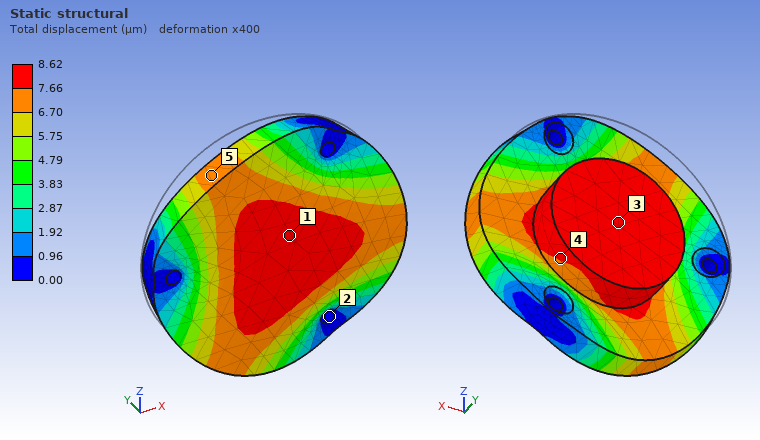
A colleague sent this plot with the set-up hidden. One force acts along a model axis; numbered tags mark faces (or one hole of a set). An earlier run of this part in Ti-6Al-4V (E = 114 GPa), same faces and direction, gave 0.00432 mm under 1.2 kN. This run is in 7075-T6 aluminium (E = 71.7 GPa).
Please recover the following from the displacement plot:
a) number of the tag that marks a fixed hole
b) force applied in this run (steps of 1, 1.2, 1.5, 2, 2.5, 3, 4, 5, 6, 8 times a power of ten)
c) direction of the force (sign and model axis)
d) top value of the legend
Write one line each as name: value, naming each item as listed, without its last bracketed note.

number of the tag that marks a fixed hole: 2
force applied in this run: 1.5 kN
direction of the force: -Y
top value of the legend: 8.62 µm
